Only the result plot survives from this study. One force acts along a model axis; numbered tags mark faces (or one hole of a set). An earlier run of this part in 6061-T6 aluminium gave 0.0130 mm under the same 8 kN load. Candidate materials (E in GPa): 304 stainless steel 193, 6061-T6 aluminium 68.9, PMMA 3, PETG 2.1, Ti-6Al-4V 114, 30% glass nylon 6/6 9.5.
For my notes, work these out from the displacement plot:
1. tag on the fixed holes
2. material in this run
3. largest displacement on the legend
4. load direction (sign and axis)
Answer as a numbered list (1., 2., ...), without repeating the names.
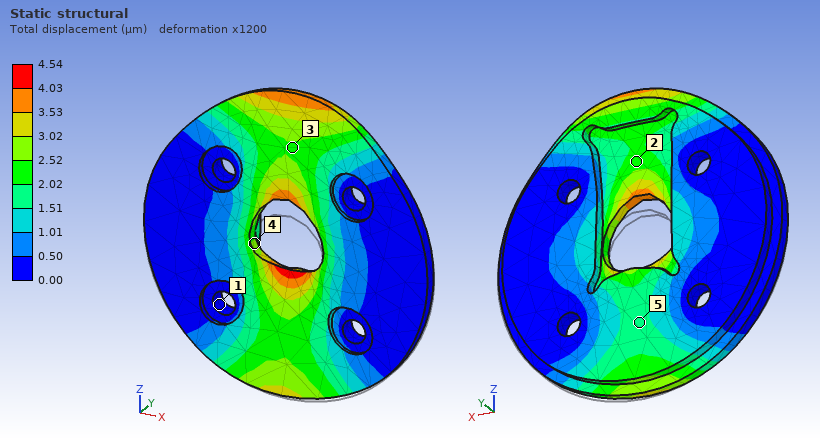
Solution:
1. 1
2. 304 stainless steel
3. 4.54 µm
4. +Z
